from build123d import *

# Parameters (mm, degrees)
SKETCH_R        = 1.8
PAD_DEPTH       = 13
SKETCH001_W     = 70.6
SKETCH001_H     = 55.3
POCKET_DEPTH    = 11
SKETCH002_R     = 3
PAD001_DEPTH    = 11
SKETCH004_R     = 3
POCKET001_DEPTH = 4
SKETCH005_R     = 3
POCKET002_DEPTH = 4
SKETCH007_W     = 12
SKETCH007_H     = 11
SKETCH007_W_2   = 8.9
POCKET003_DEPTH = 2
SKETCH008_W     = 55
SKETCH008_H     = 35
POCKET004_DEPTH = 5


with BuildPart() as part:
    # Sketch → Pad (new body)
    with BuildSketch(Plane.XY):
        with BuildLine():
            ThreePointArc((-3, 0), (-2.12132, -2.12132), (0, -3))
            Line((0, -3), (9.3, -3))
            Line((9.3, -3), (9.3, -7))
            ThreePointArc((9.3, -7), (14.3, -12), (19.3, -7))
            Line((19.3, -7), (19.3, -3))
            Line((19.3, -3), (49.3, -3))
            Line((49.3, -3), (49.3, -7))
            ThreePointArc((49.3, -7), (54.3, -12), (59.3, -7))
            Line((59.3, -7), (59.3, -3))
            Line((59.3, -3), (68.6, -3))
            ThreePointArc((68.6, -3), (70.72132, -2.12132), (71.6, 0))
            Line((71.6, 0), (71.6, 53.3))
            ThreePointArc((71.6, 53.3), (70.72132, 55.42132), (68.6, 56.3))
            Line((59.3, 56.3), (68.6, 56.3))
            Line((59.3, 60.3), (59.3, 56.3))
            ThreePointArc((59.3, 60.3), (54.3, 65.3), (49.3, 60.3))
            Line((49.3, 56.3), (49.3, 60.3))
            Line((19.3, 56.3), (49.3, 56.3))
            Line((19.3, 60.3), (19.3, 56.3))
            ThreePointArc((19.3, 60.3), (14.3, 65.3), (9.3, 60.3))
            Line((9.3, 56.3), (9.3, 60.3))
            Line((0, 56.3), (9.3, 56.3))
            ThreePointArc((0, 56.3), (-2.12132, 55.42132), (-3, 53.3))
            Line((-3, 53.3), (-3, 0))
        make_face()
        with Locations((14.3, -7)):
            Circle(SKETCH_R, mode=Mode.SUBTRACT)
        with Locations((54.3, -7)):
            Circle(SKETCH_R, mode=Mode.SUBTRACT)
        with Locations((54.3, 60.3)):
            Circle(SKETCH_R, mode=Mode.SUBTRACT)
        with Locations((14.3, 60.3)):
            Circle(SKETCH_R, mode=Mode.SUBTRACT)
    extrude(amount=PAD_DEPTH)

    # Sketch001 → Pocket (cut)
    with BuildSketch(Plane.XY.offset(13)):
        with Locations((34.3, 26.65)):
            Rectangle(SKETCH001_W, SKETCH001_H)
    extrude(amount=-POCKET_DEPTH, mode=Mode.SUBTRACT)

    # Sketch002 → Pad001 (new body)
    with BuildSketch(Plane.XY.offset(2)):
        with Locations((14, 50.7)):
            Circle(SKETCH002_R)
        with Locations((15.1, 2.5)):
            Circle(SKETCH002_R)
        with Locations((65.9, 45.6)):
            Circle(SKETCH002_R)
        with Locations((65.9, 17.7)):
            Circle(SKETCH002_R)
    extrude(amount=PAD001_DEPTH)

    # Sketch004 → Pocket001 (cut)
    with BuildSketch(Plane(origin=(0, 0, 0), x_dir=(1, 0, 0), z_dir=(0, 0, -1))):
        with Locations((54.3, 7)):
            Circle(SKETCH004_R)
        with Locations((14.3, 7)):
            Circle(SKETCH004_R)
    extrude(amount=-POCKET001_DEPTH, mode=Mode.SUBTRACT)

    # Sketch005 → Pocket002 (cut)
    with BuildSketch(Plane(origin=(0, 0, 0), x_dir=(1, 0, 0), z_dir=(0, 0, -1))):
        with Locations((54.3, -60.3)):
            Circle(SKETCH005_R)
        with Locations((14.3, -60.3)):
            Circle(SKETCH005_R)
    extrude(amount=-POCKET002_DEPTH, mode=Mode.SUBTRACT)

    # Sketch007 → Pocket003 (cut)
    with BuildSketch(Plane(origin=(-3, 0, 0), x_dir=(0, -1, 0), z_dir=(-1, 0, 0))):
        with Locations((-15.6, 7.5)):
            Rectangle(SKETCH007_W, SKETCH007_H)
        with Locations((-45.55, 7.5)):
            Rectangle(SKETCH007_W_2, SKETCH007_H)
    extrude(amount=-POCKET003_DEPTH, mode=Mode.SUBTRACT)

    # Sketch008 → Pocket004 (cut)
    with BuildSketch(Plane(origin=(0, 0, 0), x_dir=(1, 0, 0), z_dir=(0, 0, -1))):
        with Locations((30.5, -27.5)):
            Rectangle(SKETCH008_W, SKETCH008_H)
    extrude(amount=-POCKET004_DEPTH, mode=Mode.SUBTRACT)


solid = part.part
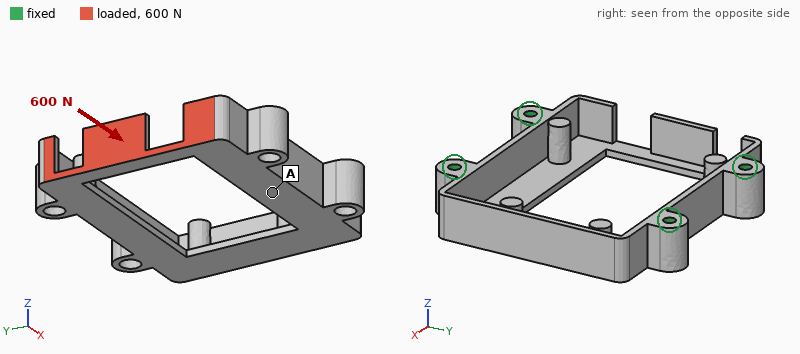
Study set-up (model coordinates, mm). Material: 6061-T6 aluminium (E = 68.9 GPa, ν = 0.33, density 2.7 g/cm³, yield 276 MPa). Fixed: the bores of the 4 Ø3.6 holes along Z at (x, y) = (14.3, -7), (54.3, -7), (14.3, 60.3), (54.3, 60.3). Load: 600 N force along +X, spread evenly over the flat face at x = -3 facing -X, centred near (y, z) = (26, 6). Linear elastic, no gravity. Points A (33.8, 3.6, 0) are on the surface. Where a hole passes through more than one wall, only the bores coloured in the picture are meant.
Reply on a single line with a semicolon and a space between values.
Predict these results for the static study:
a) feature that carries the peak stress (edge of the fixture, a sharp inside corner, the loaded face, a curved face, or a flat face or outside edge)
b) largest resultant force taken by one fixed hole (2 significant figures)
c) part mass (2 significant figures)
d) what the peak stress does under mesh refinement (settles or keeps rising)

a sharp inside corner; 290 N; 40 g; keeps rising
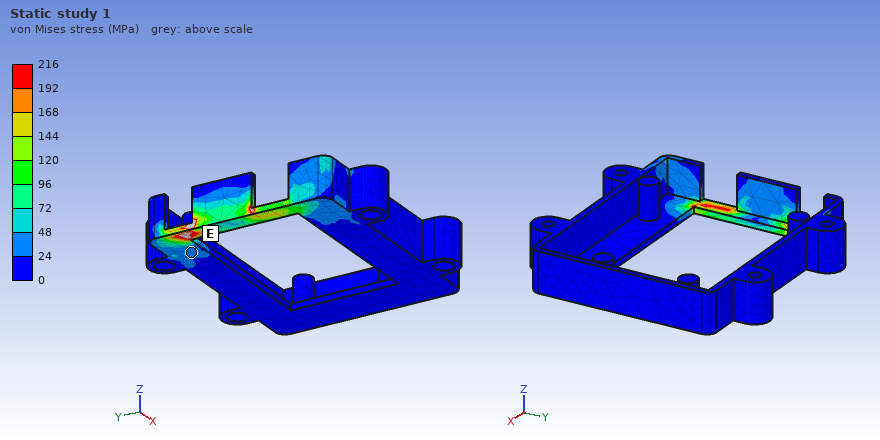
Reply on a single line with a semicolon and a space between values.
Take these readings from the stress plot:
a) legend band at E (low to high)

24 to 48 MPa
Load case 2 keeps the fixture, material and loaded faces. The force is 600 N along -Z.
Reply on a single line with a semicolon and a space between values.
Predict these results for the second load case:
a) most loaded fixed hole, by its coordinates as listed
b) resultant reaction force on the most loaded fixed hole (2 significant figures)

(14.3, -7); 460 N
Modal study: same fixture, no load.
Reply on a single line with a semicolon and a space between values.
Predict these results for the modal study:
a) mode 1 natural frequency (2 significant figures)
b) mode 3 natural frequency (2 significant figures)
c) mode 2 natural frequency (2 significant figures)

3500 Hz; 5200 Hz; 4200 Hz
